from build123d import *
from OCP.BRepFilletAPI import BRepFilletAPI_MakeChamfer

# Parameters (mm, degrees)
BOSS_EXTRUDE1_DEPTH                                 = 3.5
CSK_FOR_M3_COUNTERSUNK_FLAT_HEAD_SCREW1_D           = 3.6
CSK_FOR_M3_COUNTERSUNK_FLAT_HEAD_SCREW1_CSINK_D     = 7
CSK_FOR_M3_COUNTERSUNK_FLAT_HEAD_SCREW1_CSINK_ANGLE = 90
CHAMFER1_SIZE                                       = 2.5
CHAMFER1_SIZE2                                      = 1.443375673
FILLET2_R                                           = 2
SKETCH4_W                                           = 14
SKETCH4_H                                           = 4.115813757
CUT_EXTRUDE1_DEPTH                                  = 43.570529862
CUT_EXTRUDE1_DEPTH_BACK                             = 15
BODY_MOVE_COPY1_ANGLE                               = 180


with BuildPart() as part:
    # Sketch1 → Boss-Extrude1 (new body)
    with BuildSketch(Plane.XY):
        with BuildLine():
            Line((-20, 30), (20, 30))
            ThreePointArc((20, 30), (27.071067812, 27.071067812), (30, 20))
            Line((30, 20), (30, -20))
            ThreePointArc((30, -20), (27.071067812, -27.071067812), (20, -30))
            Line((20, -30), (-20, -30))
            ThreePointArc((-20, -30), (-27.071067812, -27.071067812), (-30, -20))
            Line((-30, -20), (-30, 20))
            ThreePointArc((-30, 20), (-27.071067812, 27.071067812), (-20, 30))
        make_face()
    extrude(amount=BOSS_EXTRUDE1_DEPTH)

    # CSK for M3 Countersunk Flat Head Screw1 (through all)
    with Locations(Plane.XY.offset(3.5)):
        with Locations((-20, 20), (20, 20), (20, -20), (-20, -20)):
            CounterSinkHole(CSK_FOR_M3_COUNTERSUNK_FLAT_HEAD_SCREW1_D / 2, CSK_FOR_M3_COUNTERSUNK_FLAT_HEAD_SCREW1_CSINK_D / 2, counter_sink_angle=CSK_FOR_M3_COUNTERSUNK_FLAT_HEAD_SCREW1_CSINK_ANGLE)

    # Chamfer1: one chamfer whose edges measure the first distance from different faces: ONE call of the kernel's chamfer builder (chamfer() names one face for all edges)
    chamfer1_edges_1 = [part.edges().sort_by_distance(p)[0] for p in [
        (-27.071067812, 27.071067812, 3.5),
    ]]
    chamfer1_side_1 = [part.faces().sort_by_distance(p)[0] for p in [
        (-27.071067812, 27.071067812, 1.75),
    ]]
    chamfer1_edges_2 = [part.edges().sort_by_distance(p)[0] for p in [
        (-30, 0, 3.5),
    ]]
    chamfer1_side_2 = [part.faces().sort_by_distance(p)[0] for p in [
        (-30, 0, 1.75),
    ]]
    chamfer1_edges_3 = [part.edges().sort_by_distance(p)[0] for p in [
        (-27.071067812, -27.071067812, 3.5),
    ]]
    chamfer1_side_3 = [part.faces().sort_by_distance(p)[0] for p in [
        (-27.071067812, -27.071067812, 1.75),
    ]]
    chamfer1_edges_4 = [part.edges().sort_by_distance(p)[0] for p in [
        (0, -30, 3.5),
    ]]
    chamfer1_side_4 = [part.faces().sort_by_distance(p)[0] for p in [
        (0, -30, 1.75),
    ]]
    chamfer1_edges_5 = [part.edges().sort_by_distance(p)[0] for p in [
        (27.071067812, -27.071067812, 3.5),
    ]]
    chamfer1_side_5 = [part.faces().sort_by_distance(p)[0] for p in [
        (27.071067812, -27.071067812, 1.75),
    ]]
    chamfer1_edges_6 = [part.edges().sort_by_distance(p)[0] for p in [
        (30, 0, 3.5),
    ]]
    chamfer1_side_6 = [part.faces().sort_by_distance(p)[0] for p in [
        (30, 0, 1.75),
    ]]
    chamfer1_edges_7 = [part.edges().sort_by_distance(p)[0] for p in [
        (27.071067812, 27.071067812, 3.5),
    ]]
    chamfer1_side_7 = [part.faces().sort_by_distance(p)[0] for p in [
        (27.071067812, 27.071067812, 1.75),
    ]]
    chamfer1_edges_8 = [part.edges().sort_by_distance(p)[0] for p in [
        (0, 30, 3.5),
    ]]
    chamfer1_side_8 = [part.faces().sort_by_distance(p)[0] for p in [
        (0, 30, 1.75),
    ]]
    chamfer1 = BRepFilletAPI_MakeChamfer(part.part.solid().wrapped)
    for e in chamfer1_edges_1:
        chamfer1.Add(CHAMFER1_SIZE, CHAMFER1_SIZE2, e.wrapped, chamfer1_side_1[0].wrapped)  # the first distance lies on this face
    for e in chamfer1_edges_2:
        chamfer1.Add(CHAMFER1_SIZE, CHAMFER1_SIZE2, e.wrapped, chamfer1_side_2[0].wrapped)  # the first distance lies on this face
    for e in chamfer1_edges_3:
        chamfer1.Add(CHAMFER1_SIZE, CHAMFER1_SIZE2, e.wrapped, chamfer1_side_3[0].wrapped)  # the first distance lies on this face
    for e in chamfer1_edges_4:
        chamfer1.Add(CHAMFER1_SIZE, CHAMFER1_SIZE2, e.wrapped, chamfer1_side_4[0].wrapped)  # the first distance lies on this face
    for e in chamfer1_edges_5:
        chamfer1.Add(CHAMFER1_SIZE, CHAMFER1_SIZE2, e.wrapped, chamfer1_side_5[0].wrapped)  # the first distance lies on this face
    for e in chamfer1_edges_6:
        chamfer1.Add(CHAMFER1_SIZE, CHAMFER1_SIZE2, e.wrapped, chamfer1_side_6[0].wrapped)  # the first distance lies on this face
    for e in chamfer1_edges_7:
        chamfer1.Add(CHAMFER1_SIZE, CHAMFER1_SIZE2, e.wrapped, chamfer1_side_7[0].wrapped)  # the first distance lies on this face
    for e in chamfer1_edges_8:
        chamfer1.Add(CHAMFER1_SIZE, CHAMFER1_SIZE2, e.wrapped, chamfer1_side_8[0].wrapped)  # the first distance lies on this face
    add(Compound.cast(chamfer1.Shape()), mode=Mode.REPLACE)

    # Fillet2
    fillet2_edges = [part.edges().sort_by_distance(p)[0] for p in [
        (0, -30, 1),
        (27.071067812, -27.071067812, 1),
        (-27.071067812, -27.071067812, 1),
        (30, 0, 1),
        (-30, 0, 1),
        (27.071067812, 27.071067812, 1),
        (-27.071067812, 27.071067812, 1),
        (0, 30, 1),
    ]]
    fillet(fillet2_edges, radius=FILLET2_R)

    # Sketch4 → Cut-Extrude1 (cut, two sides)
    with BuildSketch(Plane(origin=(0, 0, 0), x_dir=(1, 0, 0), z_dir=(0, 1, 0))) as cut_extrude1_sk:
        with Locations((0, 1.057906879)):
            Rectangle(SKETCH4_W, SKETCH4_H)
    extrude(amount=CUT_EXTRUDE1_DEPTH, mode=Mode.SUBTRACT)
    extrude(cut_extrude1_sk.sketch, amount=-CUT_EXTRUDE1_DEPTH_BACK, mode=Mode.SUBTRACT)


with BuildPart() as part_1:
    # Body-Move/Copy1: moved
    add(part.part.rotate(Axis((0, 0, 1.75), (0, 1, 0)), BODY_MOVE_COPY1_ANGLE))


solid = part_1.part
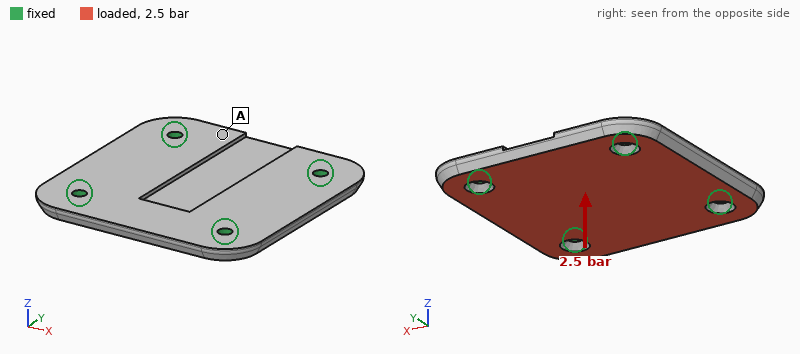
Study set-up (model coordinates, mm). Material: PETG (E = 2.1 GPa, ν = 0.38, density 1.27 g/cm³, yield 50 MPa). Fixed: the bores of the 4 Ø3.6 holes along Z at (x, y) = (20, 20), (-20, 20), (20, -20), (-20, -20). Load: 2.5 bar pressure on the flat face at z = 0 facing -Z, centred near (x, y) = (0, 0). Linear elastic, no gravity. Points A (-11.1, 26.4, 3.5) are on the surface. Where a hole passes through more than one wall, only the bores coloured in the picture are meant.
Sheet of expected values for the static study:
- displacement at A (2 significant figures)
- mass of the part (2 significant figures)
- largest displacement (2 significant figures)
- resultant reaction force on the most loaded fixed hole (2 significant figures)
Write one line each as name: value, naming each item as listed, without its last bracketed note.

displacement at A: 0.19 mm
mass of the part: 14 g
largest displacement: 0.82 mm
resultant reaction force on the most loaded fixed hole: 280 N
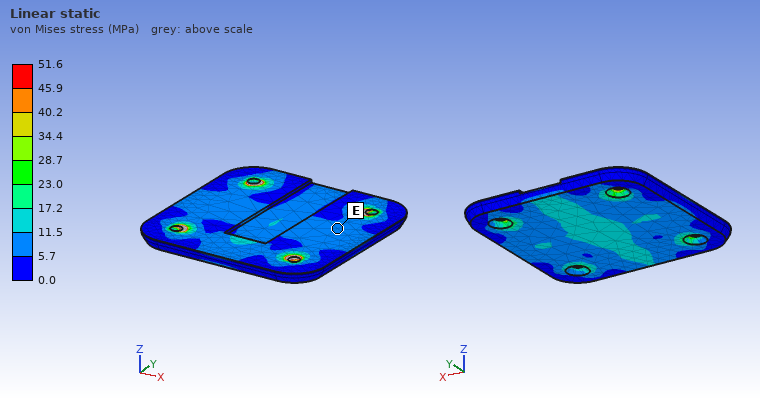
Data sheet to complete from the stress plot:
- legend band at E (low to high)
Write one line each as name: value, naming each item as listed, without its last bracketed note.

legend band at E: 5.7 to 11.5 MPa
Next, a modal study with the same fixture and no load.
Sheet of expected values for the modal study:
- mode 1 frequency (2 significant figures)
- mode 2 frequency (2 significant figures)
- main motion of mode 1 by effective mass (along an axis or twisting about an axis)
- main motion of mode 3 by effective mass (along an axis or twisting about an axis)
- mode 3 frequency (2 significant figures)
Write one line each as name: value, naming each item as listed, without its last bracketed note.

mode 1 frequency: 1800 Hz
mode 2 frequency: 2200 Hz
main motion of mode 1 by effective mass: along Z
main motion of mode 3 by effective mass: twisting about Y
mode 3 frequency: 2400 Hz
